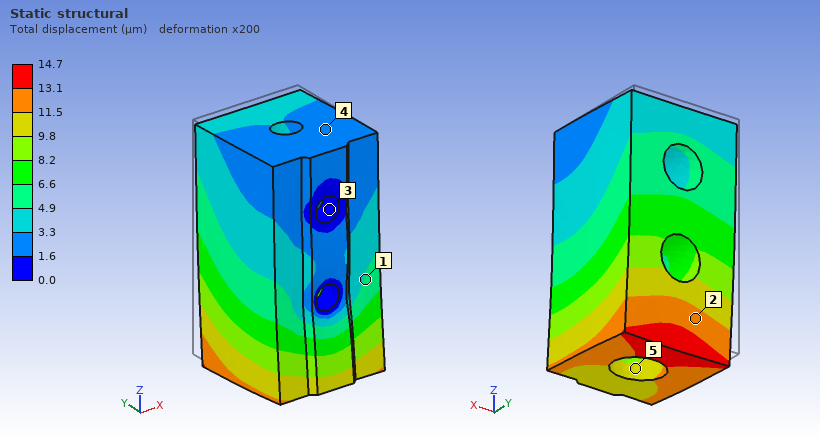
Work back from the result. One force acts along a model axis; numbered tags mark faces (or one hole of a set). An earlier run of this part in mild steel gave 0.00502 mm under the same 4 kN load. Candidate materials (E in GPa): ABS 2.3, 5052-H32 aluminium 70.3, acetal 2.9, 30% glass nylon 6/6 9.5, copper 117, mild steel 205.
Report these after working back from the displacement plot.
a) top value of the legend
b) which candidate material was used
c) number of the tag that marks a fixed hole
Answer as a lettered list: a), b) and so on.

a) 14.7 µm
b) 5052-H32 aluminium
c) 3
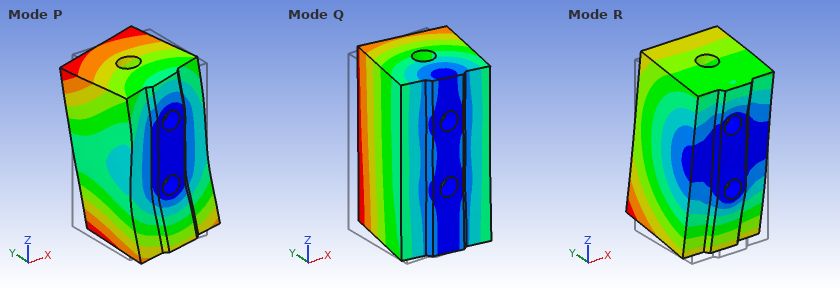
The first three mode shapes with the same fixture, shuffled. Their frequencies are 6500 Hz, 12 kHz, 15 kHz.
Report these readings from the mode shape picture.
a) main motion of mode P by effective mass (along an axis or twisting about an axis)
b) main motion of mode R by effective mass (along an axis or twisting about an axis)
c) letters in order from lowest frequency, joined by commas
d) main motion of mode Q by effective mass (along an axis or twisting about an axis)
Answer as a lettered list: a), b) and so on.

a) twisting about Y
b) along Z
c) Q, R, P
d) along X
